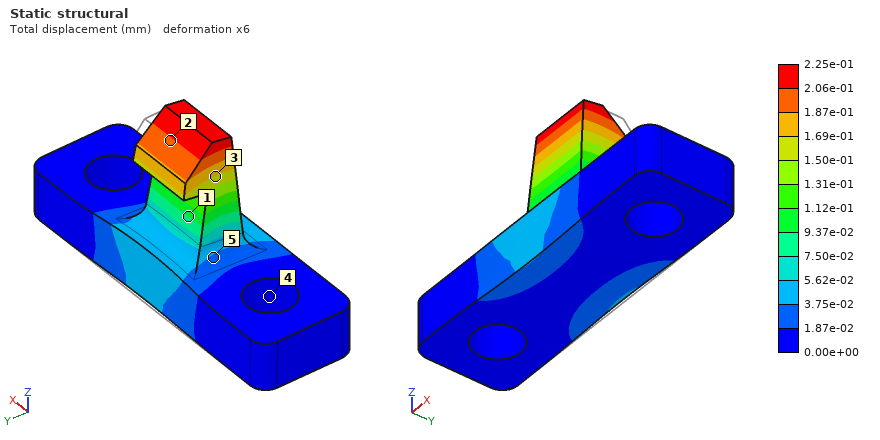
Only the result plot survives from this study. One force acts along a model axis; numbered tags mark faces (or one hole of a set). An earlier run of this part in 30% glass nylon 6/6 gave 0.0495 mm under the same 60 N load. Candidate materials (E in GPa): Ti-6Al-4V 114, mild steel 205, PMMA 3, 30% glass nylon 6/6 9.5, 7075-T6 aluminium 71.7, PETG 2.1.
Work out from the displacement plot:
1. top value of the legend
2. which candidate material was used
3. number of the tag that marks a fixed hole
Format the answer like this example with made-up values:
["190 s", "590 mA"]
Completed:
["2.25e-01 mm", "PETG", "4"]
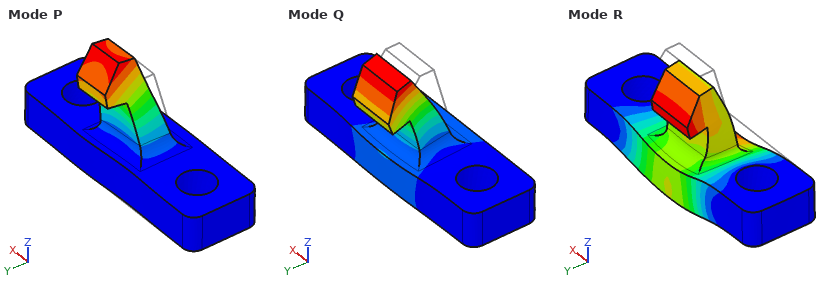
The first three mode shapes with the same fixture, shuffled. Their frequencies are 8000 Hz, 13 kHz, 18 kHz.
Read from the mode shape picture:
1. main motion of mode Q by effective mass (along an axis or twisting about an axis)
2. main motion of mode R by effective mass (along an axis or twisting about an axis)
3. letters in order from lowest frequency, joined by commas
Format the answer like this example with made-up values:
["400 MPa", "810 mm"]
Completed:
["along Y", "along Z", "Q, P, R"]
